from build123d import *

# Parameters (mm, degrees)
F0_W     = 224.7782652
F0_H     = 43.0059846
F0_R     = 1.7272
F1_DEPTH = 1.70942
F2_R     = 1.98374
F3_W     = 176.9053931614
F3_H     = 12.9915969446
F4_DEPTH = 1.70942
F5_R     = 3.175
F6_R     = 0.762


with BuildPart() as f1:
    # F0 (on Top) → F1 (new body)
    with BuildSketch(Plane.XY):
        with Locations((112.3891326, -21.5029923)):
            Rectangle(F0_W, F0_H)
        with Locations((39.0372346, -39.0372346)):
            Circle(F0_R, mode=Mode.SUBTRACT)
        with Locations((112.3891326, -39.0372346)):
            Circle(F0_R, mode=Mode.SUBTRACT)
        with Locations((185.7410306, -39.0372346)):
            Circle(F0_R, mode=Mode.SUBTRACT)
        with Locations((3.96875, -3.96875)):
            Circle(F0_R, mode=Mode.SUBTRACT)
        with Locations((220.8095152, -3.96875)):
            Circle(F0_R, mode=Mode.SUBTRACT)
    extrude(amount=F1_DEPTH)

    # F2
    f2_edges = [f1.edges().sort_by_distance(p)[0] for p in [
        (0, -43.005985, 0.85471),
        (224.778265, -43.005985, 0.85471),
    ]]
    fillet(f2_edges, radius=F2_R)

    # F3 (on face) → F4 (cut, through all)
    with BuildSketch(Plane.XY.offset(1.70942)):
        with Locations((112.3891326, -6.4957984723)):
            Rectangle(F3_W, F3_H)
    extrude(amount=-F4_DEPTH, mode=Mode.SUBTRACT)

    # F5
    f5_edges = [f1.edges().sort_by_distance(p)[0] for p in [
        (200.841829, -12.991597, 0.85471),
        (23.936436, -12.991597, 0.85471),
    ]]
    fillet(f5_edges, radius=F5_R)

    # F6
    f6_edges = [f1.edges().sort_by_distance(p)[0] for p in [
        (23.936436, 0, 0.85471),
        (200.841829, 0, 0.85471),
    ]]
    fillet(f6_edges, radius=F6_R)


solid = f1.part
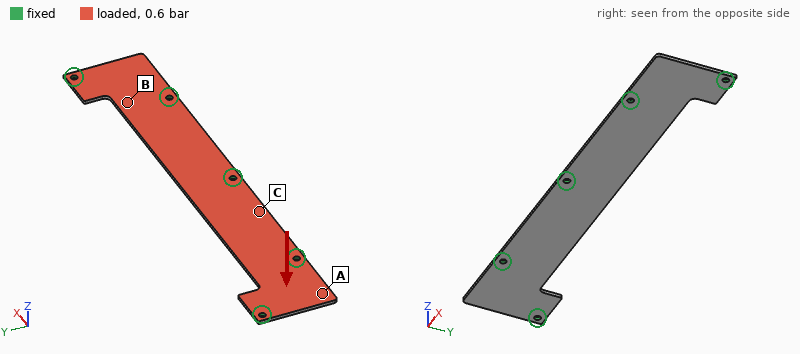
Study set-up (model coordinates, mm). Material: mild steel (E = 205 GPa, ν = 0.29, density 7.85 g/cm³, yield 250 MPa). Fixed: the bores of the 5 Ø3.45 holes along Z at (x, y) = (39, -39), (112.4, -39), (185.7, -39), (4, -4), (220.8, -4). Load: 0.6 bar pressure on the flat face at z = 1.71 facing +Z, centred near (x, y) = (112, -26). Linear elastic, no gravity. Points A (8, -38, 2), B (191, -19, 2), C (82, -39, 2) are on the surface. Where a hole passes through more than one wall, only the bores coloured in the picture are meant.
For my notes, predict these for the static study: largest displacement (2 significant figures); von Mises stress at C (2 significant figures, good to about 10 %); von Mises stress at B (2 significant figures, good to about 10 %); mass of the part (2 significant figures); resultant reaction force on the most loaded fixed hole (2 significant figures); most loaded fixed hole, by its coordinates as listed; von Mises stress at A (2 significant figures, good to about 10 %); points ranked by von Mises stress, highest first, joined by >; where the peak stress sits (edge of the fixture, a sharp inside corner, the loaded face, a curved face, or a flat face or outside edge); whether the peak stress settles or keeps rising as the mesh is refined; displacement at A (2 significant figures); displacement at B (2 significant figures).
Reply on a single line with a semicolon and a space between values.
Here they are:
0.13 mm; 24 MPa; 31 MPa; 98 g; 140 N; (112.4, -39); 10 MPa; B > C > A; edge of the fixture; keeps rising; 0.028 mm; 0.029 mm
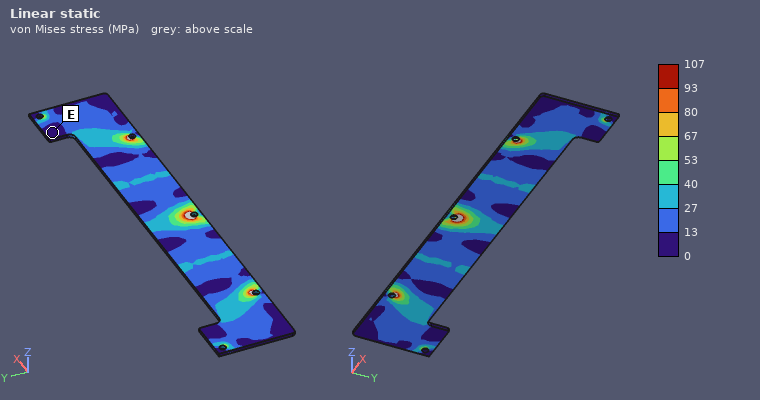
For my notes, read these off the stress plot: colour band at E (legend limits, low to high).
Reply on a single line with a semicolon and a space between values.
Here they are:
0 to 13 MPa
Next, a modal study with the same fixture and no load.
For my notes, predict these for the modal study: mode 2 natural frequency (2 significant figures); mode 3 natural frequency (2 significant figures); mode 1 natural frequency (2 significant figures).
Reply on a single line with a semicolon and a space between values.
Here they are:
1200 Hz; 1800 Hz; 1200 Hz
